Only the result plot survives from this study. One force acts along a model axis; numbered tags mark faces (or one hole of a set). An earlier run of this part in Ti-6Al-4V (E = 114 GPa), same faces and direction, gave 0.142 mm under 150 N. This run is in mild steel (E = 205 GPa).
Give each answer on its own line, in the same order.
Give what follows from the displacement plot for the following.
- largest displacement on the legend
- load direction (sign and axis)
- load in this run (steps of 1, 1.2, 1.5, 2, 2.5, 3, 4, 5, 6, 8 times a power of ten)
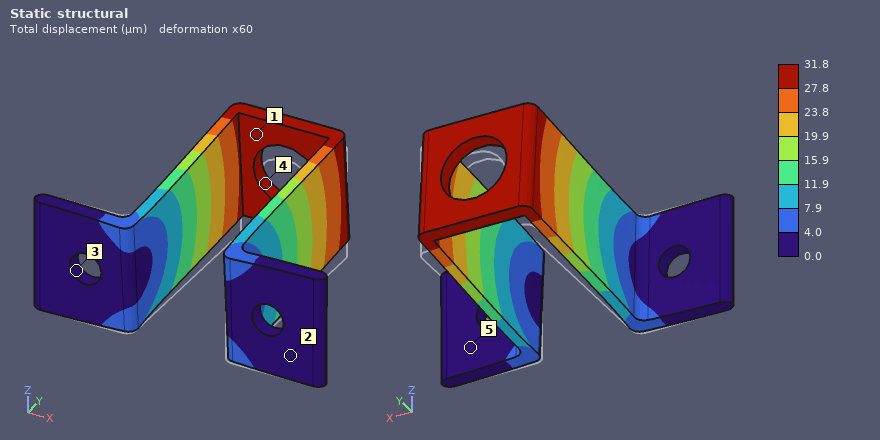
31.8 µm
+Z
60 N
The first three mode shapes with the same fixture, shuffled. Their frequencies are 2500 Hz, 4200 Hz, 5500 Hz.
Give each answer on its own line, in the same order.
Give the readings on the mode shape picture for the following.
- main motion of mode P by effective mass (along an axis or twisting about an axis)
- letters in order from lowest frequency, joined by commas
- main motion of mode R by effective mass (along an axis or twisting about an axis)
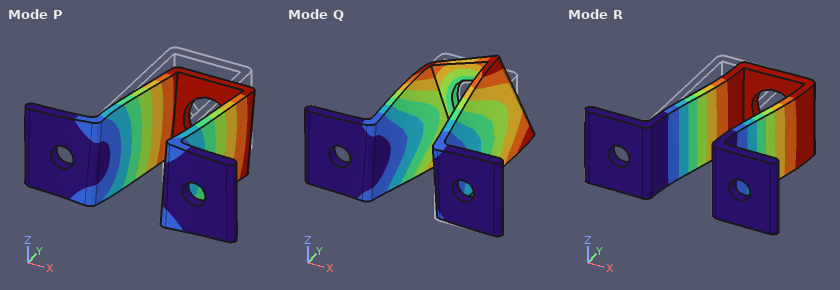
along Z
R, P, Q
along X
